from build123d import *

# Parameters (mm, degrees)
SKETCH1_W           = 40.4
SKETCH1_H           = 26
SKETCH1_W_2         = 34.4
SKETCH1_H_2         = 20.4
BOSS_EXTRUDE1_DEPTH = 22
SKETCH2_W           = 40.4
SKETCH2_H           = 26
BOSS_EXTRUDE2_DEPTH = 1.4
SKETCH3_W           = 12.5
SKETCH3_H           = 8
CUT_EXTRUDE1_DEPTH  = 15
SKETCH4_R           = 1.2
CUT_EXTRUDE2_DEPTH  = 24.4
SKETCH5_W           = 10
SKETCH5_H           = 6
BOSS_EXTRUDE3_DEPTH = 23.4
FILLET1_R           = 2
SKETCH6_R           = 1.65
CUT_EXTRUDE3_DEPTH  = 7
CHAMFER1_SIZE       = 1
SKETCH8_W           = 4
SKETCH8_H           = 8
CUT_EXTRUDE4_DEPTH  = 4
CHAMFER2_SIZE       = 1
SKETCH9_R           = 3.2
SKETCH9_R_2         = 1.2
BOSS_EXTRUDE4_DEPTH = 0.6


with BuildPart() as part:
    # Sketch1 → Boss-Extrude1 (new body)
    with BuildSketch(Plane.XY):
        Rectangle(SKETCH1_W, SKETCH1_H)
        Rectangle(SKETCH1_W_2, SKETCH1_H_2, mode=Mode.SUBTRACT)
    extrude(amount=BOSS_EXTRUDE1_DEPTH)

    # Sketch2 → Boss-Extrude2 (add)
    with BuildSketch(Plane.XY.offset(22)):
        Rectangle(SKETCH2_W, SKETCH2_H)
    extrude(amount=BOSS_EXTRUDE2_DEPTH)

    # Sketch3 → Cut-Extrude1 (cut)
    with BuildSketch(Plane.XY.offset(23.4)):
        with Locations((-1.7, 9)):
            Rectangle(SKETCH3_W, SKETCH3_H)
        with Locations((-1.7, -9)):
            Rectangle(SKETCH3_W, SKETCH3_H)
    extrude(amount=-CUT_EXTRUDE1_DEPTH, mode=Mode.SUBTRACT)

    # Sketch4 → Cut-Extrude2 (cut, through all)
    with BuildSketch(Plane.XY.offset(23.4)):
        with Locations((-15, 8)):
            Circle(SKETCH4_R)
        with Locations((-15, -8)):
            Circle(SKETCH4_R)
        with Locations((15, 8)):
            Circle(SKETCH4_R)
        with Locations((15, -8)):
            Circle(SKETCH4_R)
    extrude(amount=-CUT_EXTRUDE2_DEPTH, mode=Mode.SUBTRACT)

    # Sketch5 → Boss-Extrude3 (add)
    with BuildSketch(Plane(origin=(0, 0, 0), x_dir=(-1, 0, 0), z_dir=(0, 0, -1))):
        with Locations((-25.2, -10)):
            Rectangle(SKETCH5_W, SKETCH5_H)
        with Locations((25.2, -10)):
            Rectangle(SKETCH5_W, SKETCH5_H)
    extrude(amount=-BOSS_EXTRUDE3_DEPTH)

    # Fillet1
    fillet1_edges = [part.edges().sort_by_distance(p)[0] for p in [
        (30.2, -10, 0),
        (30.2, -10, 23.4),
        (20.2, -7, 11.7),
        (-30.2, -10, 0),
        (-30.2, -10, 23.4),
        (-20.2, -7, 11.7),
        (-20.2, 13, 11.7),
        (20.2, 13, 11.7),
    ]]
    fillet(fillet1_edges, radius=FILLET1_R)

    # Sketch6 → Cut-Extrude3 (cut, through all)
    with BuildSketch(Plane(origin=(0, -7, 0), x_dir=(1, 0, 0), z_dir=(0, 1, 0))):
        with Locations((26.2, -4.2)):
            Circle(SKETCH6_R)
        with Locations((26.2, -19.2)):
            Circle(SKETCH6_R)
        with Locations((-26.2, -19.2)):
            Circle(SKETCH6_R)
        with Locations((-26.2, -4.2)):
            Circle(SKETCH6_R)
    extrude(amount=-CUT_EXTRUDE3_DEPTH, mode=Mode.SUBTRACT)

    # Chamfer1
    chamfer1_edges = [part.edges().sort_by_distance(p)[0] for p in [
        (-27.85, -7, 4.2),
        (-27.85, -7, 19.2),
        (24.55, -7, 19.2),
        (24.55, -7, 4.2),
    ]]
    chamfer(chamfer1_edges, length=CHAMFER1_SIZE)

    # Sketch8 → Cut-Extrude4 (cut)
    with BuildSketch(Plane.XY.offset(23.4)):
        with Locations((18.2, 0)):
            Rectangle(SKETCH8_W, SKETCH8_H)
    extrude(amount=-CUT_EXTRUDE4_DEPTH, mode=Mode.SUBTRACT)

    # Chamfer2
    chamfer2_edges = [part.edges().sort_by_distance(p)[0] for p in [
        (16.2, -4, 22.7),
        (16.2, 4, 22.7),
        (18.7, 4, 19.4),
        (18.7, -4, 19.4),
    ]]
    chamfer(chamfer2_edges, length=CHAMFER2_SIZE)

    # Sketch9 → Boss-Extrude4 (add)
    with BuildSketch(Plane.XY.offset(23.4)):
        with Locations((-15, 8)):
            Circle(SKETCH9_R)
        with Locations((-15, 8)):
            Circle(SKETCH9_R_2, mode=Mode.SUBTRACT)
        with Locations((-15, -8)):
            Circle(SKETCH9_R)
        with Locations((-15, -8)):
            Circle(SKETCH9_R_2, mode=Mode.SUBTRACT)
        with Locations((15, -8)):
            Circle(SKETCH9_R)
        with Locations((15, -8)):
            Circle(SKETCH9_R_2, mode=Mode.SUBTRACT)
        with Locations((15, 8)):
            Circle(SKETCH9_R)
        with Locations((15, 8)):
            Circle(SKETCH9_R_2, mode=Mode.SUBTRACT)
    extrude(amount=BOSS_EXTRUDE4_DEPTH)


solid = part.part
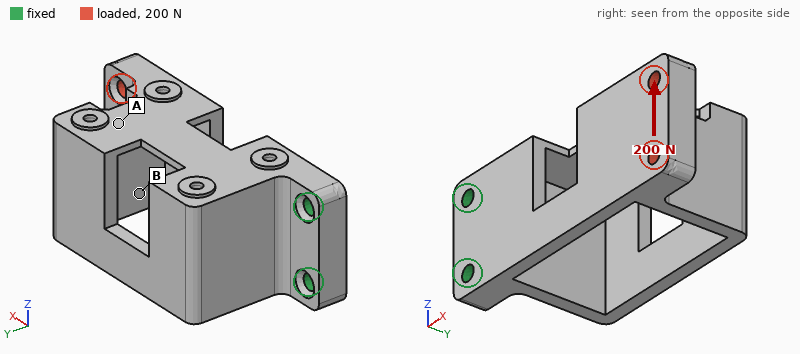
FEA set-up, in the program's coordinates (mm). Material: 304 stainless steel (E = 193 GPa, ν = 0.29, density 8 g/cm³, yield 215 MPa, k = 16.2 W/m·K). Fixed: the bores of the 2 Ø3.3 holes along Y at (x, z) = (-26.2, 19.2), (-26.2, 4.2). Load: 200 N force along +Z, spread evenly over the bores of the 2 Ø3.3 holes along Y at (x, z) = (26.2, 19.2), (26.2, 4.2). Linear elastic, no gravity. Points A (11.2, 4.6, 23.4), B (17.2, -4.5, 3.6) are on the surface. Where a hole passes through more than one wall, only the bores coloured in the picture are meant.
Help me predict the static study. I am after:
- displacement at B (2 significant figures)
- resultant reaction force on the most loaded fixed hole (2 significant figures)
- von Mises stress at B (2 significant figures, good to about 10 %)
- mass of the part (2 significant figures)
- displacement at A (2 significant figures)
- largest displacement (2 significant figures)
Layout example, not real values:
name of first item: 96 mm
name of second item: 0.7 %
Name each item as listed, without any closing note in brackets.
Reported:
displacement at B: 33 µm
resultant reaction force on the most loaded fixed hole: 640 N
von Mises stress at B: 17 MPa
mass of the part: 83 g
displacement at A: 23 µm
largest displacement: 50 µm
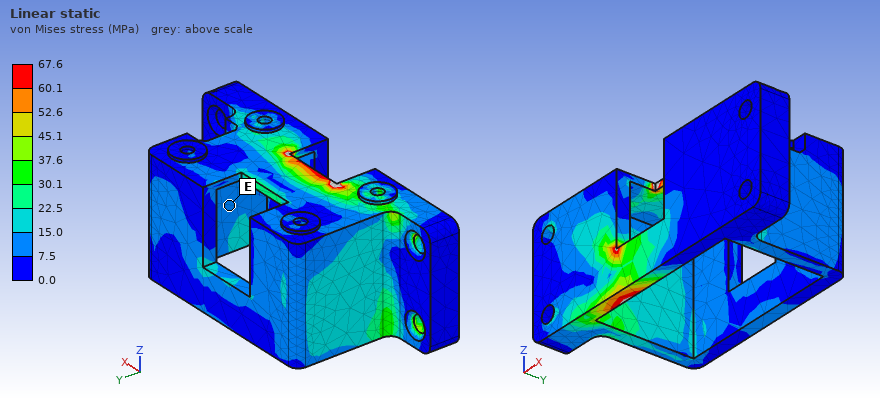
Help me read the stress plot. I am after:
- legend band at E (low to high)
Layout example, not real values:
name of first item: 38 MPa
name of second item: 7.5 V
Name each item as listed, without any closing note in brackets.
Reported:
legend band at E: 7.5 to 15.0 MPa
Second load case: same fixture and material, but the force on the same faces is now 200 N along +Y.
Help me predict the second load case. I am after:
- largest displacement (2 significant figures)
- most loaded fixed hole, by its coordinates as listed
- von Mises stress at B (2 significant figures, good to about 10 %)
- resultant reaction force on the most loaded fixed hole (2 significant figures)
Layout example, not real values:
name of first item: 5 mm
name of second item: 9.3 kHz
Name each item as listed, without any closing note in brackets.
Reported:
largest displacement: 0.17 mm
most loaded fixed hole, by its coordinates as listed: (-26.2, 4.2)
von Mises stress at B: 50 MPa
resultant reaction force on the most loaded fixed hole: 110 N
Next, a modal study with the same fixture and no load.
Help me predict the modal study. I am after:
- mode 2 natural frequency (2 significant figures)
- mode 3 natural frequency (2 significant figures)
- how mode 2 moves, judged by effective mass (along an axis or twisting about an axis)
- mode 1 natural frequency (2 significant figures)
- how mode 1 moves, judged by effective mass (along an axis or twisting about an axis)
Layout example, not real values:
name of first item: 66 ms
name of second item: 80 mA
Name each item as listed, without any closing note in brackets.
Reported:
mode 2 natural frequency: 2100 Hz
mode 3 natural frequency: 3400 Hz
how mode 2 moves, judged by effective mass: along Z
mode 1 natural frequency: 1000 Hz
how mode 1 moves, judged by effective mass: along Y
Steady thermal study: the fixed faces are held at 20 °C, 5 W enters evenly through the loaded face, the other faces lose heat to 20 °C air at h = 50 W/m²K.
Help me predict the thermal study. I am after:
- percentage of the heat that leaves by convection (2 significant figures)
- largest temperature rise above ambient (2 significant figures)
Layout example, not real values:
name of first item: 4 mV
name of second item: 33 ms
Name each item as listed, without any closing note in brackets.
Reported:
percentage of the heat that leaves by convection: 95 %
largest temperature rise above ambient: 50 K
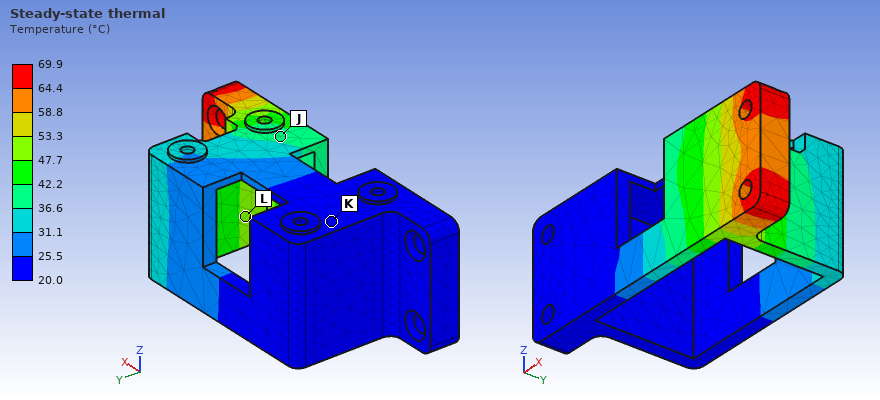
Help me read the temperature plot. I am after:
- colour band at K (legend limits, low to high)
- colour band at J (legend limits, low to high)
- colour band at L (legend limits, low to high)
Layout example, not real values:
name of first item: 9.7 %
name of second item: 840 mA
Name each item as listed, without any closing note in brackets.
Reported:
colour band at K: 20.0 to 25.5 °C
colour band at J: 36.6 to 42.2 °C
colour band at L: 47.7 to 53.3 °C
